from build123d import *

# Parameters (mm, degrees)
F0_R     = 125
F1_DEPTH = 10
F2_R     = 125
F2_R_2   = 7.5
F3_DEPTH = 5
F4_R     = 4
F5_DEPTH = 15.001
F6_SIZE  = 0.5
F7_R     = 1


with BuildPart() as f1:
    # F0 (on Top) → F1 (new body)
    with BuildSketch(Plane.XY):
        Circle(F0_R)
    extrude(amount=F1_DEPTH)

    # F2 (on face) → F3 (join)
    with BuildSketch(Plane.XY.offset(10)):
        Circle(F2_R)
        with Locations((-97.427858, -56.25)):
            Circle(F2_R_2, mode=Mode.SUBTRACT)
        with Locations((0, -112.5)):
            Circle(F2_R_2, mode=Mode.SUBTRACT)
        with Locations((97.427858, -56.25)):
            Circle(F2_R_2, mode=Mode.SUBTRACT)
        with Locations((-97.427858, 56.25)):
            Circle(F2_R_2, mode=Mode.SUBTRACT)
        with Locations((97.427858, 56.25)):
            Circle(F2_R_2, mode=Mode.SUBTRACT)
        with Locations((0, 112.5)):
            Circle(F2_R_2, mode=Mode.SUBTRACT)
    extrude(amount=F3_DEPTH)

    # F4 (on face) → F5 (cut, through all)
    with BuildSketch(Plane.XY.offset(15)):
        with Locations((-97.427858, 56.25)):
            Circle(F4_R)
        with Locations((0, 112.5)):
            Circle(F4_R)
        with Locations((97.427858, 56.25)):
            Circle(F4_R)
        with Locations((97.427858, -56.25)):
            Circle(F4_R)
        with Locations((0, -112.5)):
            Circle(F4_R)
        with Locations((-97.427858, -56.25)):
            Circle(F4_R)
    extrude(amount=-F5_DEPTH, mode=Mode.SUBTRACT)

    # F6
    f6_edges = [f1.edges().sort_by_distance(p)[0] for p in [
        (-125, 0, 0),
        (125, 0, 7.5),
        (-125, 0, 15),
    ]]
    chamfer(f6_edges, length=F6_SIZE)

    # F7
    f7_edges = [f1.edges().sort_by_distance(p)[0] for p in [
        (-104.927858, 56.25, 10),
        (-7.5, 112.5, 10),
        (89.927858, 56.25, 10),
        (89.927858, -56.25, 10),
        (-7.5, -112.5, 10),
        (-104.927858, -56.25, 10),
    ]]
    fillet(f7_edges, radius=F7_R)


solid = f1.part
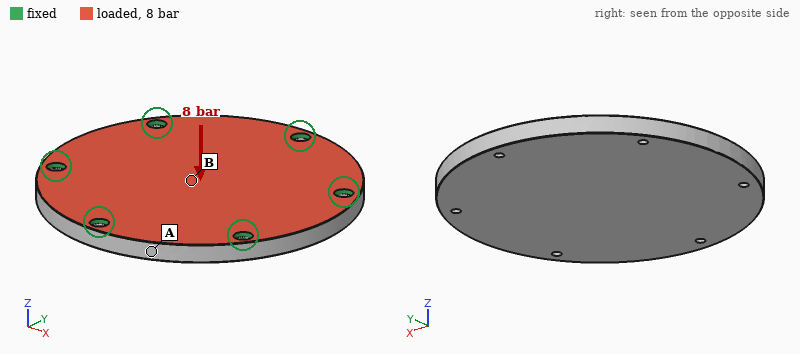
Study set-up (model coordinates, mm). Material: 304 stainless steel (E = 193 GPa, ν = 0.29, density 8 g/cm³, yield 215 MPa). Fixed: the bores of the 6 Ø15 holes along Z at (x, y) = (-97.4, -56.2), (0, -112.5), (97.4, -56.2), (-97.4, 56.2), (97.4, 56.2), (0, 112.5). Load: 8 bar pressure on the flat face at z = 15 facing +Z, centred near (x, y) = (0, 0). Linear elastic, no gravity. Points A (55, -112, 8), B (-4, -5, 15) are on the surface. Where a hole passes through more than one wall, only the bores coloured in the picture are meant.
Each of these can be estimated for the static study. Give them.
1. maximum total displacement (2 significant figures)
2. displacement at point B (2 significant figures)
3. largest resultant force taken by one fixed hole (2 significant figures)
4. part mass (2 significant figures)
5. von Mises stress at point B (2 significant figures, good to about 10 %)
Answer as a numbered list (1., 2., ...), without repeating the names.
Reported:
1. 62 µm
2. 62 µm
3. 8.2 kN
4. 5.8 kg
5. 26 MPa
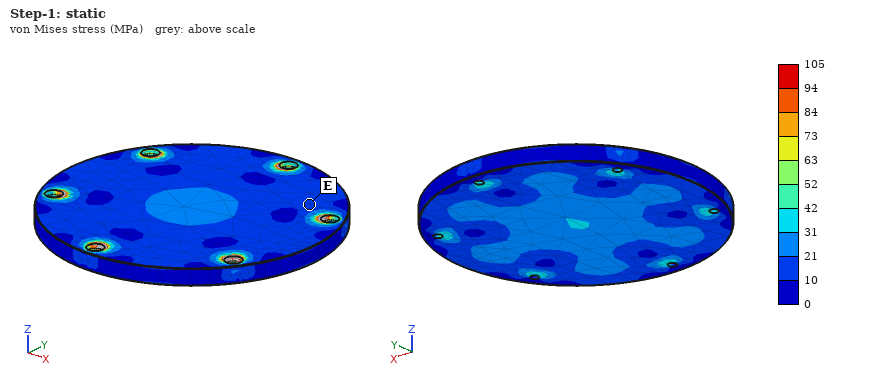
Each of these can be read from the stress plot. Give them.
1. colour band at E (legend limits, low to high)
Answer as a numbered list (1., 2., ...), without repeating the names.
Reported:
1. 10 to 21 MPa
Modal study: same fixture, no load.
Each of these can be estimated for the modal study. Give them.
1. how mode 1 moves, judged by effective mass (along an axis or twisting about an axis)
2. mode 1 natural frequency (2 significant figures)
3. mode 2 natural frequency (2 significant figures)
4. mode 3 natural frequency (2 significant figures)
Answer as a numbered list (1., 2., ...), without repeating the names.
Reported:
1. along Z
2. 2000 Hz
3. 4100 Hz
4. 4100 Hz
